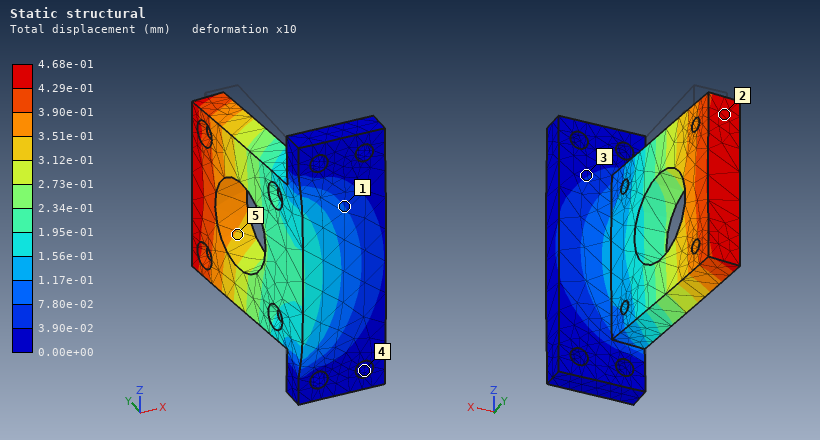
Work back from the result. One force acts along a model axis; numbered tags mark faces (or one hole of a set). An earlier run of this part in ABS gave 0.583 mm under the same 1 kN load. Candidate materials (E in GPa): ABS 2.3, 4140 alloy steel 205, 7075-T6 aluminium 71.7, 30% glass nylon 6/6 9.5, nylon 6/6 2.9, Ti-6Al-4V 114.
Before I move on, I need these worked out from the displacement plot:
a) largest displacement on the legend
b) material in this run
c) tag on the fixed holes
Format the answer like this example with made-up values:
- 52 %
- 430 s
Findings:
- 4.68e-01 mm
- nylon 6/6
- 4
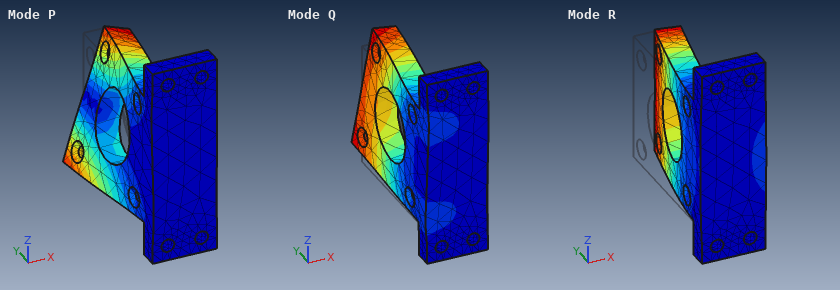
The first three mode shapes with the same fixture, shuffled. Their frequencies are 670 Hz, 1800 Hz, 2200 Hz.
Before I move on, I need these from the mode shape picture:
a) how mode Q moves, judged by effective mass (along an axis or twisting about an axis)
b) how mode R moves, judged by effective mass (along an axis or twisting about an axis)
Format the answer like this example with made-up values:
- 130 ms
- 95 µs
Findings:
- along Z
- along X
